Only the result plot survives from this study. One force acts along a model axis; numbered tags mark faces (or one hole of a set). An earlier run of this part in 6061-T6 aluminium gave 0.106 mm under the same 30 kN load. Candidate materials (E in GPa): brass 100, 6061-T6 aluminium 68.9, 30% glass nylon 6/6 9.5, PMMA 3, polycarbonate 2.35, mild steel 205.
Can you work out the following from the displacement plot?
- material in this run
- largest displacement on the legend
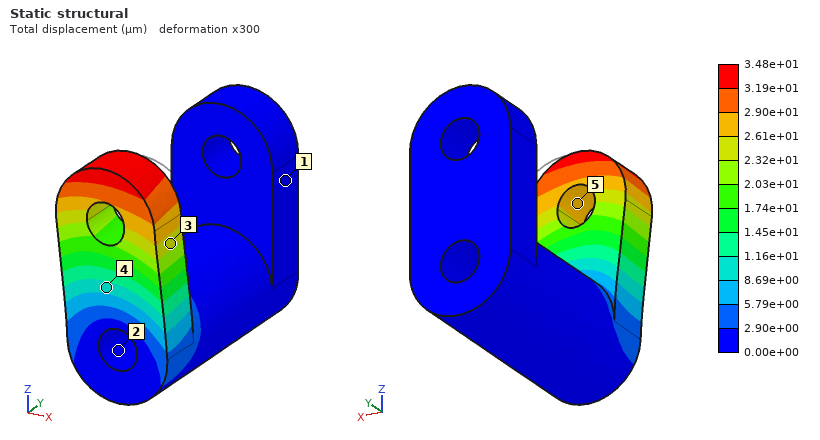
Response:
mild steel
3.48e+01 µm
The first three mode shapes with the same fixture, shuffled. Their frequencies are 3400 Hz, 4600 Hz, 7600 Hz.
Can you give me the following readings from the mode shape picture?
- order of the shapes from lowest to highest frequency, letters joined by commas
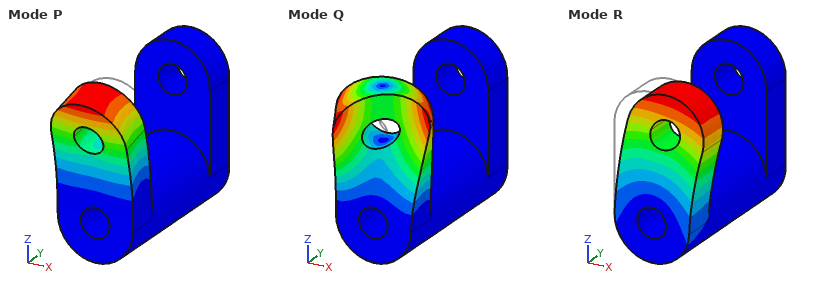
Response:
P, R, Q
